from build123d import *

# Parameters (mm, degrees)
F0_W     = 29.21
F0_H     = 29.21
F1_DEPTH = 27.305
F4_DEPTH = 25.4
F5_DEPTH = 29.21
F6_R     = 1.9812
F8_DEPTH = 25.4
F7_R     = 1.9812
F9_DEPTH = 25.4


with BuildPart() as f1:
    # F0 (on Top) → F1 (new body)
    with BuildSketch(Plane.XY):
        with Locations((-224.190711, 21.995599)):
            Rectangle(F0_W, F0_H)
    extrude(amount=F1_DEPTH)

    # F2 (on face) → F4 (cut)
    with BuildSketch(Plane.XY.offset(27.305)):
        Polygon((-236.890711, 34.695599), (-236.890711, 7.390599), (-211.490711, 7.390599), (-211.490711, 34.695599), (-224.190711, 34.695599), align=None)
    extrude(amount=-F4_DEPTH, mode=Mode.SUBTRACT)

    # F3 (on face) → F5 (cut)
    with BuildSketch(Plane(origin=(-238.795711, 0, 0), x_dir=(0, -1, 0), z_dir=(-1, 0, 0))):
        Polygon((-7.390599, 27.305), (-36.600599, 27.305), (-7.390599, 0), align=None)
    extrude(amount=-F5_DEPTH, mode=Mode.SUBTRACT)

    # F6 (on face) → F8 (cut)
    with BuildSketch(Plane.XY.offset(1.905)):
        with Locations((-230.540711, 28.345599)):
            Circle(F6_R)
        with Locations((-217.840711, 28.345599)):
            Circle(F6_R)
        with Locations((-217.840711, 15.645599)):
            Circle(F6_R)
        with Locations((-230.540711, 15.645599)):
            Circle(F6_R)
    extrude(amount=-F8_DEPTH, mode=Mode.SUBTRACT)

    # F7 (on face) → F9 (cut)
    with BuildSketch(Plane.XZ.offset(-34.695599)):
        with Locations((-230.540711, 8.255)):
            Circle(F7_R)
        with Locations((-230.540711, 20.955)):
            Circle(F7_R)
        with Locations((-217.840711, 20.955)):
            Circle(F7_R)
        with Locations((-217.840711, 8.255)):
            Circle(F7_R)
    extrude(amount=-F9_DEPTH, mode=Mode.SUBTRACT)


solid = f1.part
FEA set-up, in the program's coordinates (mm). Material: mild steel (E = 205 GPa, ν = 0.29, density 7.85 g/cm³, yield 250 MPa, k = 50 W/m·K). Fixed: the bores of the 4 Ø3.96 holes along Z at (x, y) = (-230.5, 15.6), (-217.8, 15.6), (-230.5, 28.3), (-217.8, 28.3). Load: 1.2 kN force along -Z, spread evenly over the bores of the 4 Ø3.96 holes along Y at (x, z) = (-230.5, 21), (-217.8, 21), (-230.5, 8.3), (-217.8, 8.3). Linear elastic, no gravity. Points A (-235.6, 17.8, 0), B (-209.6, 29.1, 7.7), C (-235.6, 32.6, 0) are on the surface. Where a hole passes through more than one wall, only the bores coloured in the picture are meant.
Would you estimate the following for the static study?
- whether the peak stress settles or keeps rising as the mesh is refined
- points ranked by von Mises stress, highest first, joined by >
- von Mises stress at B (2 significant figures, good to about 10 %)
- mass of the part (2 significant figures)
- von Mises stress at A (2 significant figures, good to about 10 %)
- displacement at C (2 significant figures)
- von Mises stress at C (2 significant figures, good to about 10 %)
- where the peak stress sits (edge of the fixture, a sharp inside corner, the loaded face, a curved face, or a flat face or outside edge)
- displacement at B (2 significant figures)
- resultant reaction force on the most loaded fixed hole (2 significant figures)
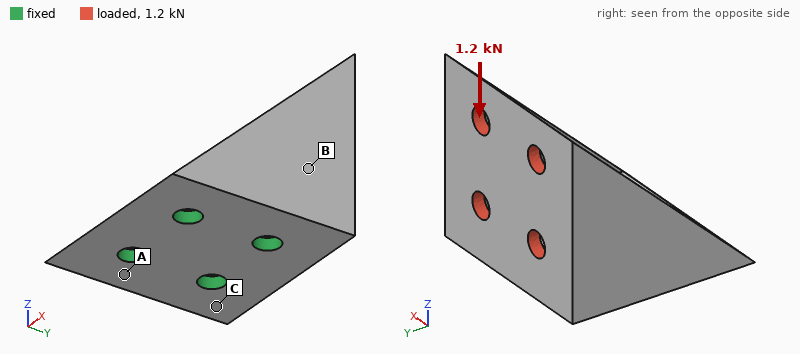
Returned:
keeps rising
C > A > B
23 MPa
30 g
40 MPa
11 µm
80 MPa
edge of the fixture
11 µm
750 N
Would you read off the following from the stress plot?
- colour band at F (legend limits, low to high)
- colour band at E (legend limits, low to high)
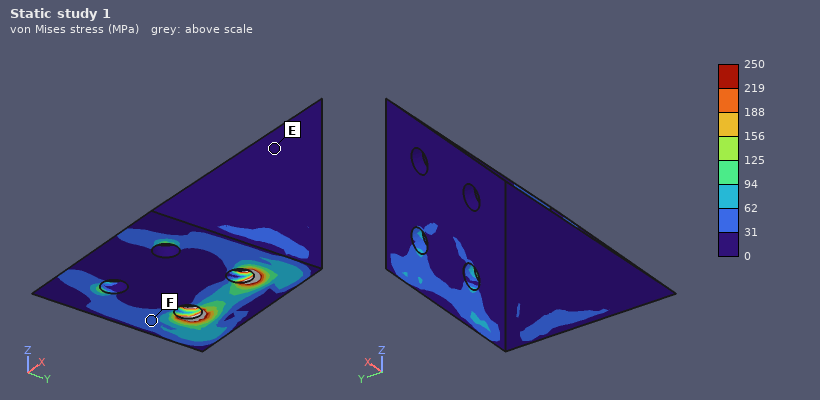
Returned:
31 to 62 MPa
0 to 31 MPa
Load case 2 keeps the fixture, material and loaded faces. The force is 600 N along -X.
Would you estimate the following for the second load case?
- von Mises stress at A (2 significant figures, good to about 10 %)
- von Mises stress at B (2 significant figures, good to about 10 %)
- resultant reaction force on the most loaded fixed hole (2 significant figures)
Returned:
39 MPa
21 MPa
620 N
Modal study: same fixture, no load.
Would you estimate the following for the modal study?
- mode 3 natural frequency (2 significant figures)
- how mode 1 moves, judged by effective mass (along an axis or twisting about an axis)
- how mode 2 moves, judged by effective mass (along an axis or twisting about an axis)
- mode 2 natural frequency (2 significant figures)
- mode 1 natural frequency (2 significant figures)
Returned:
11 kHz
along X
along Y
5800 Hz
5200 Hz
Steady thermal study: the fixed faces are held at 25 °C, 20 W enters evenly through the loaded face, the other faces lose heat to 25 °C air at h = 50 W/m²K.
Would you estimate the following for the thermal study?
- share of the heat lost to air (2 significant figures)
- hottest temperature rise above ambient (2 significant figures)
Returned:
31 %
79 K
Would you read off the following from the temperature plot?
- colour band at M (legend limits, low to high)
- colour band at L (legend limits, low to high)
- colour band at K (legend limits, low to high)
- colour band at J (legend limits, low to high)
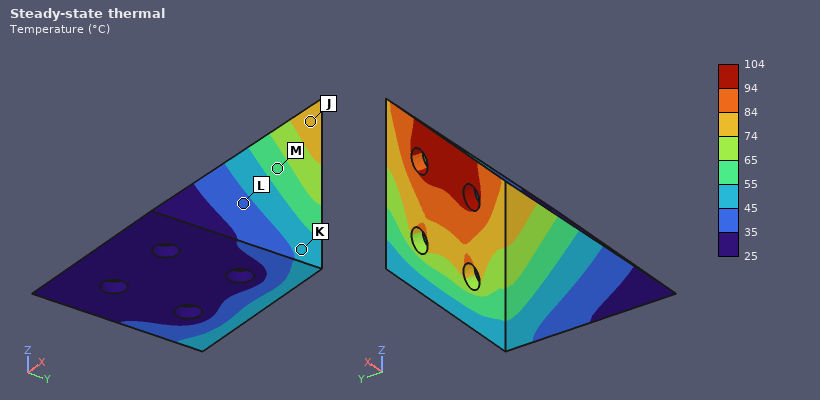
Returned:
55 to 65 °C
35 to 45 °C
45 to 55 °C
74 to 84 °C
